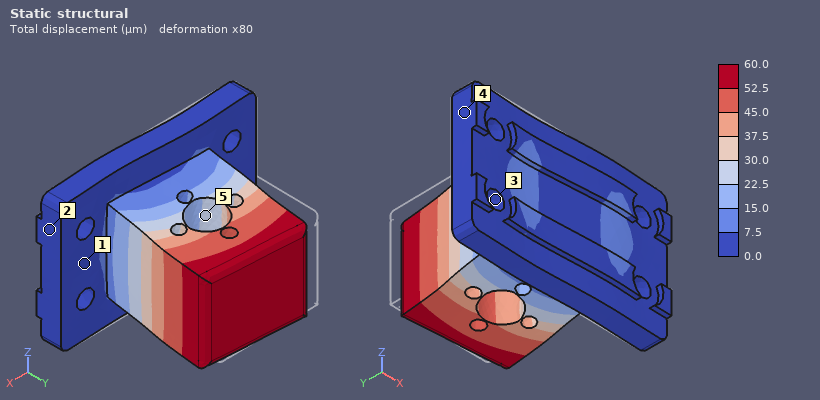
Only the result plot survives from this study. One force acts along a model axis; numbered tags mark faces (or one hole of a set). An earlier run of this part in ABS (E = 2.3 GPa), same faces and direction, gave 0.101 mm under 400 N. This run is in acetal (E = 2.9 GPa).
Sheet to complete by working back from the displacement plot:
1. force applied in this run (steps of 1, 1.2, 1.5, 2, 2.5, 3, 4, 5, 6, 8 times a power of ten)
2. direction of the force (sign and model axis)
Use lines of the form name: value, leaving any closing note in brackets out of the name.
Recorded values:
force applied in this run: 300 N
direction of the force: +X
